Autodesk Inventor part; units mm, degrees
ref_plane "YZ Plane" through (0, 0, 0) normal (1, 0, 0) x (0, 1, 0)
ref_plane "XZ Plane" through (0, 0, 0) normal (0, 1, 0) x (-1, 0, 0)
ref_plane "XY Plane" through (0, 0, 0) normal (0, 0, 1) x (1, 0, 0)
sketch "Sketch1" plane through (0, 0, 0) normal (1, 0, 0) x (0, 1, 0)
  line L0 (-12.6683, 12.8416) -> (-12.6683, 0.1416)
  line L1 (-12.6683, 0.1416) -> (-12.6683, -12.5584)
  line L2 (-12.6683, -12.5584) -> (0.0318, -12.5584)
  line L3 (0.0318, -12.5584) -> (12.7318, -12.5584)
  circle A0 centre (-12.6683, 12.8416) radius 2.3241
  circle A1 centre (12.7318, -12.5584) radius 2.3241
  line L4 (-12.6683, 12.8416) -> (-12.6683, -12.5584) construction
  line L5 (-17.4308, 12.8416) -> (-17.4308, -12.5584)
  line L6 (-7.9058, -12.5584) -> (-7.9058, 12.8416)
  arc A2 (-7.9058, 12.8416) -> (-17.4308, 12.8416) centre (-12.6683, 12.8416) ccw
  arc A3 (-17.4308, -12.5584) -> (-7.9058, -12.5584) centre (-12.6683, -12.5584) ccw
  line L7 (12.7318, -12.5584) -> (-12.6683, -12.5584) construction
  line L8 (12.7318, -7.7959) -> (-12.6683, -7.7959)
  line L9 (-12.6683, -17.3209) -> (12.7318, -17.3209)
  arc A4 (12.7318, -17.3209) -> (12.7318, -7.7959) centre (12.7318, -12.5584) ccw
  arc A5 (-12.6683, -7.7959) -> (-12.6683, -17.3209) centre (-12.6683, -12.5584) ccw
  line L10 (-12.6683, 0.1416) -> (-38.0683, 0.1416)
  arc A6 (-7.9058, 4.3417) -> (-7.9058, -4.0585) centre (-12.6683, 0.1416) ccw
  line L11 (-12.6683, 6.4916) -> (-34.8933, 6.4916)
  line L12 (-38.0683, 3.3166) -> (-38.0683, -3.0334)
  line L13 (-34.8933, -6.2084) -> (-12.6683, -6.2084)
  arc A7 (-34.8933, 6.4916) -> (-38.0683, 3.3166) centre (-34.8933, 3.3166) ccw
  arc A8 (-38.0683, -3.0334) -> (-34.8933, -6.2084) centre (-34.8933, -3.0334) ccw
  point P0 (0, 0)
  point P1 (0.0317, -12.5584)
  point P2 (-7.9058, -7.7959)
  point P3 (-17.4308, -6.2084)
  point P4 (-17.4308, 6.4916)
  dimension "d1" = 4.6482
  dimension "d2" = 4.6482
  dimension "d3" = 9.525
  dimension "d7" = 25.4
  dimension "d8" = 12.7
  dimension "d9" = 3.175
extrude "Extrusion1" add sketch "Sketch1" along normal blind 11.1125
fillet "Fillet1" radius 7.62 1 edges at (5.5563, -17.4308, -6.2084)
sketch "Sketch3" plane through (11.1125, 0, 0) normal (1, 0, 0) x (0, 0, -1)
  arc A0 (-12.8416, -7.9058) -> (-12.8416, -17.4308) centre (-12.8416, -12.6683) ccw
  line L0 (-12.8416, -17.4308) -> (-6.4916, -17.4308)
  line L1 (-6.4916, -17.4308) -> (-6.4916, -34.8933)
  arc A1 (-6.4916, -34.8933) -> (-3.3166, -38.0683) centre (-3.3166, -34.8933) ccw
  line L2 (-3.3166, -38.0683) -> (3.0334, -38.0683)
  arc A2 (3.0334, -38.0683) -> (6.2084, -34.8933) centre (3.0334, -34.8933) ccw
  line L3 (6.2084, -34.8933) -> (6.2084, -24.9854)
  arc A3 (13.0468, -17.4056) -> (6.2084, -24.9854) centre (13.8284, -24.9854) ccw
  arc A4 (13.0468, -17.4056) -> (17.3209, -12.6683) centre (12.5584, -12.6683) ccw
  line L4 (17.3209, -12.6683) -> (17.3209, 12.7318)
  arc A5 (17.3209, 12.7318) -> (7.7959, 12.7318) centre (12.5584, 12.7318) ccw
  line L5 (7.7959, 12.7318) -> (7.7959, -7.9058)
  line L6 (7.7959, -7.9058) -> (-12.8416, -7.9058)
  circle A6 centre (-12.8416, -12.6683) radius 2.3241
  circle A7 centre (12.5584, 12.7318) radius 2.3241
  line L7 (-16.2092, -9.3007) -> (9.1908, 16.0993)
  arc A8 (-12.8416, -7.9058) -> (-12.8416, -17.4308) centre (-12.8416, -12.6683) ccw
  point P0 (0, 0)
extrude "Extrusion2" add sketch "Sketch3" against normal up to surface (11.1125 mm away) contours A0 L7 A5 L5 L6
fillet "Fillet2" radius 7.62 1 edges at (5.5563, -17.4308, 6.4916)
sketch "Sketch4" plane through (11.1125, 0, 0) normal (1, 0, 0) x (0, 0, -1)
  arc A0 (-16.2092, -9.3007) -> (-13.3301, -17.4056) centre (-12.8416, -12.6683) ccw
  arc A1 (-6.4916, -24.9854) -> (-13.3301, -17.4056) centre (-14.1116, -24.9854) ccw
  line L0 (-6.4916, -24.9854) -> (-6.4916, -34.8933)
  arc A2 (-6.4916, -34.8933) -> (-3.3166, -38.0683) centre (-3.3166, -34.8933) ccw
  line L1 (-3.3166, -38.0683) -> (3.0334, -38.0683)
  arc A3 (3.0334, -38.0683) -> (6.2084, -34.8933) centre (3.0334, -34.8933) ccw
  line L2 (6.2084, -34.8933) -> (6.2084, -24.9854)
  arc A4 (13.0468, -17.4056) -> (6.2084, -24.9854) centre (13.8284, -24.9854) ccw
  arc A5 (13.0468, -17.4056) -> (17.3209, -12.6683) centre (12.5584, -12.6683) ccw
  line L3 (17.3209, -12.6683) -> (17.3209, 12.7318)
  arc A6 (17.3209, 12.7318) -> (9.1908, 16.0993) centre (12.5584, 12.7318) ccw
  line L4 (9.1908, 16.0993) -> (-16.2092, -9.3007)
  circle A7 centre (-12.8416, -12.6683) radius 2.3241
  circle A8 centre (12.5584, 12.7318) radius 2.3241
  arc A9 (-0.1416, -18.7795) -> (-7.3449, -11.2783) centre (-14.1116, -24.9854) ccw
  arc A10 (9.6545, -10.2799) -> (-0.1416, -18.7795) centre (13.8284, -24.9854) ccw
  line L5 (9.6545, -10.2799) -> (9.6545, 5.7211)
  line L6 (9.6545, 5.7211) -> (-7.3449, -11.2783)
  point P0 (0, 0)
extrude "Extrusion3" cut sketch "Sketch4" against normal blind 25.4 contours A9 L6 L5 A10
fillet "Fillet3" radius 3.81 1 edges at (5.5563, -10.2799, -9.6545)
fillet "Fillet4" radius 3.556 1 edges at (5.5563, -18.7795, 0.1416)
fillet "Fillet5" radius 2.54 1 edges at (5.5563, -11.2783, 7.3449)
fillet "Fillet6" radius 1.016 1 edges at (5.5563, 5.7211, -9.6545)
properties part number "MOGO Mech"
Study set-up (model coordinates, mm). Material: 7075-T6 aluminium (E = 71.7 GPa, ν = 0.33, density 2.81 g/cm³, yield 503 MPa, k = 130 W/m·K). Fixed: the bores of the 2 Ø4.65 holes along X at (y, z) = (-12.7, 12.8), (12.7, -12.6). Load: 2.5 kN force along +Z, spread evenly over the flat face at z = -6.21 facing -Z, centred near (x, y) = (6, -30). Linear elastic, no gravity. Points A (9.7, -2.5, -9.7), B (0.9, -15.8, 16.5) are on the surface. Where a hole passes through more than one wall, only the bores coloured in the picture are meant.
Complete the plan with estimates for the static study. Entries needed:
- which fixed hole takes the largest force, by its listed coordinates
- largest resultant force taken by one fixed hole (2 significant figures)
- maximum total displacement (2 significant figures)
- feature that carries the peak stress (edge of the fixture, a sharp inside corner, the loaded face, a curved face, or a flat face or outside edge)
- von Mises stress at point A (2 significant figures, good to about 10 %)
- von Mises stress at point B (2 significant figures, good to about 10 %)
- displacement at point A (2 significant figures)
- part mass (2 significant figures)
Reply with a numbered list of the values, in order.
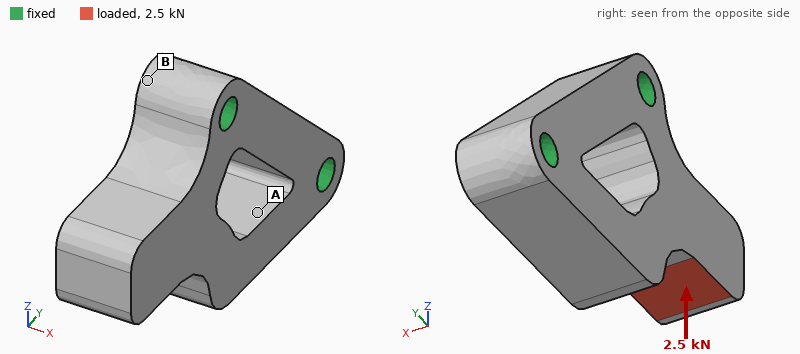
1. (-12.7, 12.8)
2. 2.8 kN
3. 49 µm
4. a curved face
5. 34 MPa
6. 9.4 MPa
7. 7.5 µm
8. 27 g
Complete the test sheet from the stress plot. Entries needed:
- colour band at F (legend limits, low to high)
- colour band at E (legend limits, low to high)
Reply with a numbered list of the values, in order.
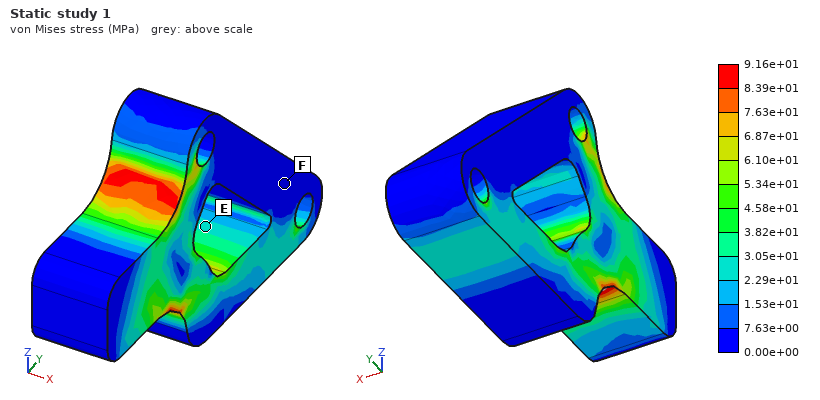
1. 0.00e+00 to 7.63e+00 MPa
2. 2.29e+01 to 3.05e+01 MPa
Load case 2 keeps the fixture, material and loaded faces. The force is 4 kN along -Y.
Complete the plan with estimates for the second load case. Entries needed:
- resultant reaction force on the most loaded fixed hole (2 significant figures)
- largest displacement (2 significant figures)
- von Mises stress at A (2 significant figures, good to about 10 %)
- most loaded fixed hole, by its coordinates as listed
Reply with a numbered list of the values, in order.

1. 3.0 kN
2. 68 µm
3. 60 MPa
4. (12.7, -12.6)
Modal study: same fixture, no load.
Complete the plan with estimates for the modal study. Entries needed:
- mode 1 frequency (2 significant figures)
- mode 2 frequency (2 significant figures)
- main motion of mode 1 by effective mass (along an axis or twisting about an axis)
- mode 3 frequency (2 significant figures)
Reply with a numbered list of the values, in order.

1. 8500 Hz
2. 15 kHz
3. along X
4. 16 kHz
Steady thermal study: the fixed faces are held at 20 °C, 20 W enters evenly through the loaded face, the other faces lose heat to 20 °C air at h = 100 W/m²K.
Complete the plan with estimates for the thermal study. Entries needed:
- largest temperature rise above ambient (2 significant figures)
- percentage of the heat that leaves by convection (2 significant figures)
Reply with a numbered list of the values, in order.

1. 26 K
2. 14 %
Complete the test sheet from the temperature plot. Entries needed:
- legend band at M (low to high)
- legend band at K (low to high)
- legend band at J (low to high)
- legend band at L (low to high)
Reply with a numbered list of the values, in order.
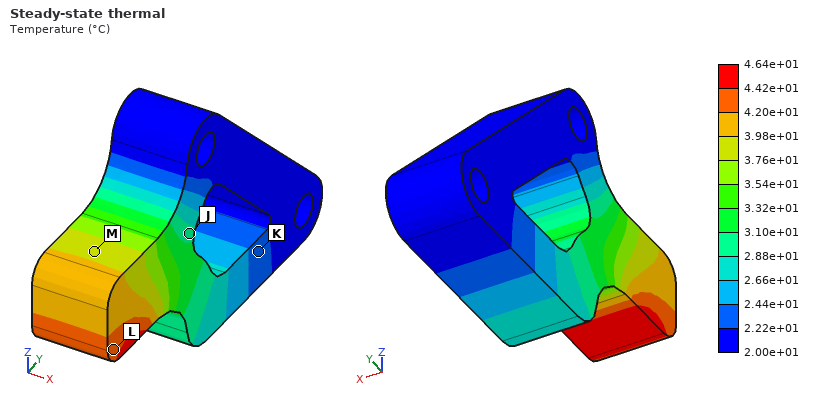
1. 3.76e+01 to 3.98e+01 °C
2. 2.22e+01 to 2.44e+01 °C
3. 2.88e+01 to 3.10e+01 °C
4. 4.20e+01 to 4.42e+01 °C
